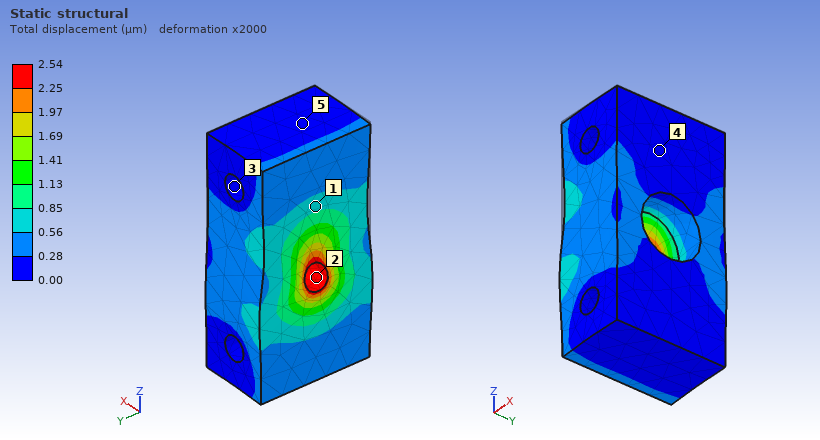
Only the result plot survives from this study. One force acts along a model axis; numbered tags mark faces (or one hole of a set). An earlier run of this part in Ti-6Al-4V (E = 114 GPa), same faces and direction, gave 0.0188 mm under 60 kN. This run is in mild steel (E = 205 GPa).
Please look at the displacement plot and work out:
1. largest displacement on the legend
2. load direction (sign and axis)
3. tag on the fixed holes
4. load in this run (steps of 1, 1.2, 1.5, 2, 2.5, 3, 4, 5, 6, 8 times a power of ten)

2.54 µm
-Z
3
15 kN
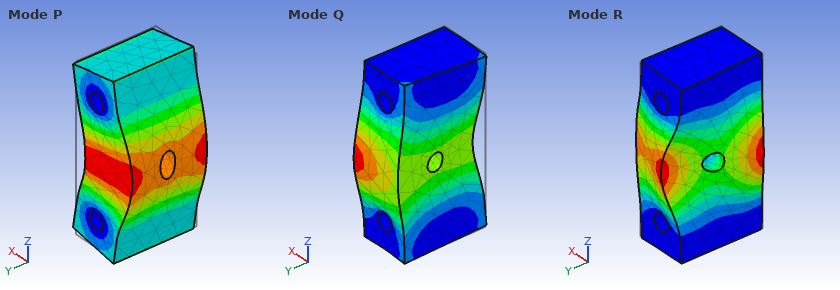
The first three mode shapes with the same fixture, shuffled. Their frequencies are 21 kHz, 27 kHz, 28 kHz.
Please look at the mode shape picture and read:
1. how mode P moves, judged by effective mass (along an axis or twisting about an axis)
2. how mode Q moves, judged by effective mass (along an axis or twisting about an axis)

along X
along Y
